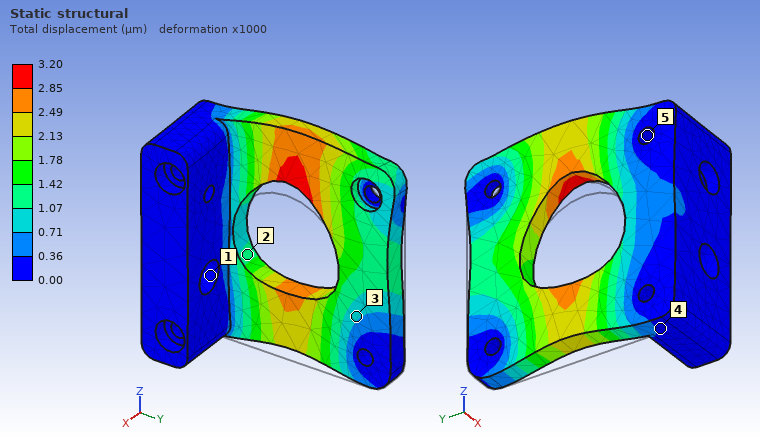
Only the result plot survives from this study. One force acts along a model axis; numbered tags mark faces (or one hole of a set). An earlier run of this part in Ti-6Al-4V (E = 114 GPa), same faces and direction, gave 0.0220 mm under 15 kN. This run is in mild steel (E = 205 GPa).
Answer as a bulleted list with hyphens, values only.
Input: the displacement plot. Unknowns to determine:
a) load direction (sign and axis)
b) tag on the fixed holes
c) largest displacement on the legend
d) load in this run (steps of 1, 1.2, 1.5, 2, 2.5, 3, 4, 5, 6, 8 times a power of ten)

- +Z
- 5
- 3.20 µm
- 4 kN
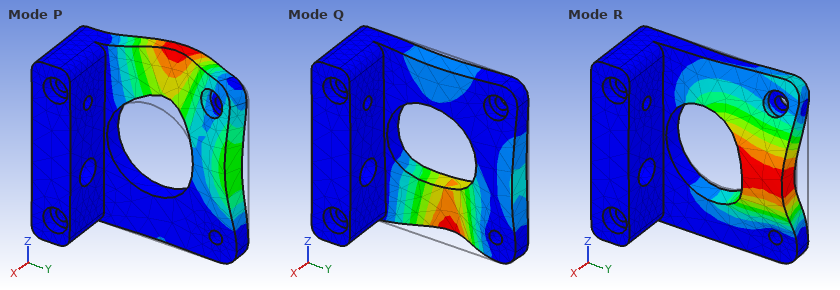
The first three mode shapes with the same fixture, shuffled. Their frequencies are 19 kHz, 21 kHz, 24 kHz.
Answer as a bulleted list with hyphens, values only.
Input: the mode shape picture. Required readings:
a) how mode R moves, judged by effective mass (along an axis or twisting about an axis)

- along X
